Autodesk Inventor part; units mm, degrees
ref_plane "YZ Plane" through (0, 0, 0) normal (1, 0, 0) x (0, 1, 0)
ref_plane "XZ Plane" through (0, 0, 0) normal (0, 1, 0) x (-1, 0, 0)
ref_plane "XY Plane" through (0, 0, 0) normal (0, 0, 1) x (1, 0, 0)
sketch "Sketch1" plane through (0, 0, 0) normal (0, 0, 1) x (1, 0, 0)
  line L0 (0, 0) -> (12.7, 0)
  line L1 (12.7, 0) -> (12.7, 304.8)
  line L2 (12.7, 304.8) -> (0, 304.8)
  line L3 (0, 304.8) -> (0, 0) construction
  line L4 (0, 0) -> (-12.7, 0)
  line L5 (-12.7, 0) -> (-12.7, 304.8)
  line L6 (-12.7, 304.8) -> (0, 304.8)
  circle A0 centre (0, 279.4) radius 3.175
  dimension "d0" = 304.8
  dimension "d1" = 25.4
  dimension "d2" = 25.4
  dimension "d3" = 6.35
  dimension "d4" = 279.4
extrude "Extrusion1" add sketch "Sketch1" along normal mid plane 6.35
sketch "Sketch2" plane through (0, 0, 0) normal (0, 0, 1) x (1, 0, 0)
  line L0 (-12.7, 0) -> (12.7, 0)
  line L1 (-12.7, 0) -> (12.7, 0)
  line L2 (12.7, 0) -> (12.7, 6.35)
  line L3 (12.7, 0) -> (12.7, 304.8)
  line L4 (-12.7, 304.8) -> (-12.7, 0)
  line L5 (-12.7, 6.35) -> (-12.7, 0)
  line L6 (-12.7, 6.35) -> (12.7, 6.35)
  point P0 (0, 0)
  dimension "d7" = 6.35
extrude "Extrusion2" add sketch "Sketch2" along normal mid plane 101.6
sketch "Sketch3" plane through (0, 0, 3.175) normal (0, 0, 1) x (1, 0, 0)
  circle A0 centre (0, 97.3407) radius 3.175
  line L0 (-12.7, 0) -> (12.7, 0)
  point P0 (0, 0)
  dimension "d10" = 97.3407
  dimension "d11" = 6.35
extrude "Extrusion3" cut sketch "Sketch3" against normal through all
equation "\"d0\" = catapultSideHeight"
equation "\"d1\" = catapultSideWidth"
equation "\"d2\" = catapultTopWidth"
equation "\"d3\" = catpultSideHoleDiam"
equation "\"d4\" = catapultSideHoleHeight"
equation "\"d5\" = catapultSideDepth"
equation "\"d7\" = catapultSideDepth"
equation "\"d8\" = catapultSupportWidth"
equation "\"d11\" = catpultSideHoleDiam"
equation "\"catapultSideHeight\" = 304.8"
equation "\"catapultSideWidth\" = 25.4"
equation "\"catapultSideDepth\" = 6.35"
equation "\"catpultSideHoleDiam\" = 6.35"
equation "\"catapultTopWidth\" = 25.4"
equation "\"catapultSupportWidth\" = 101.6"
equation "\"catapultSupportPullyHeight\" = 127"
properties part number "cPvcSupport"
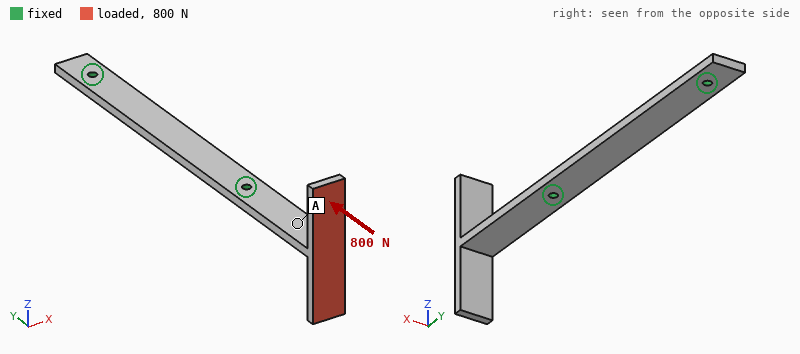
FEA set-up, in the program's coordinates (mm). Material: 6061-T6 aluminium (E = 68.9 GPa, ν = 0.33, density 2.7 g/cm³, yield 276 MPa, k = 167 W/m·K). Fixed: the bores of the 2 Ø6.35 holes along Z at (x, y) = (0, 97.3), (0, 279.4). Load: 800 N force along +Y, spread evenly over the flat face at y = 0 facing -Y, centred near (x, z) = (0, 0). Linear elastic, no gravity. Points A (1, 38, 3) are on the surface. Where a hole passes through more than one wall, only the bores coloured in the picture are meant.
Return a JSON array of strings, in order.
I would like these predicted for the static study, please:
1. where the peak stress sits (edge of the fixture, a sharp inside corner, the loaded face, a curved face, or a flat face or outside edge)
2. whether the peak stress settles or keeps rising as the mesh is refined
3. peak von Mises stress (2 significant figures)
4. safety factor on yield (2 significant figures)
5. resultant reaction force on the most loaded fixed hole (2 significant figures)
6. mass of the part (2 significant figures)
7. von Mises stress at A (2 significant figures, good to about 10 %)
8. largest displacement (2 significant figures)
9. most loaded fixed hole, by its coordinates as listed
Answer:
["the loaded face", "settles", "48 MPa", "5.8", "780 N", "170 g", "4.9 MPa", "0.17 mm", "(0, 97.3)"]
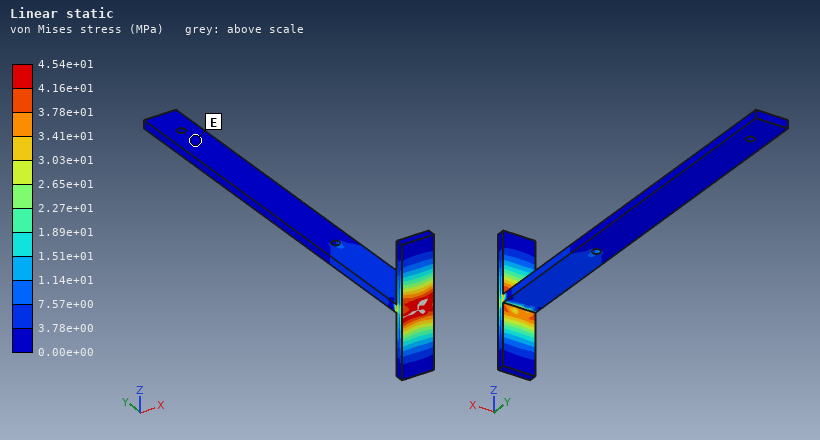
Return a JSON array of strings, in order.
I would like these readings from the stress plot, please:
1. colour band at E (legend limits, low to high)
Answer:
["0.00e+00 to 3.78e+00 MPa"]
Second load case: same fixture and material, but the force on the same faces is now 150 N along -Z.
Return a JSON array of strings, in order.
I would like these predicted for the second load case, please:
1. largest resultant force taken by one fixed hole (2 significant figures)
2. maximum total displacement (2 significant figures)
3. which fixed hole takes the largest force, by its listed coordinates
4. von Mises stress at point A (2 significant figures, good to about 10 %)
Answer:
["150 N", "1.5 mm", "(0, 97.3)", "33 MPa"]
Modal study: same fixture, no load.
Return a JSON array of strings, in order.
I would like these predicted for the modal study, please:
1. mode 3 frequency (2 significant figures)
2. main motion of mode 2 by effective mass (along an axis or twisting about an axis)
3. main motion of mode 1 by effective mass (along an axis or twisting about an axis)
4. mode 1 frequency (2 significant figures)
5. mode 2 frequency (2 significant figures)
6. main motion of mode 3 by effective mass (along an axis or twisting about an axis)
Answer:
["790 Hz", "twisting about Y", "along Z", "240 Hz", "580 Hz", "along X"]
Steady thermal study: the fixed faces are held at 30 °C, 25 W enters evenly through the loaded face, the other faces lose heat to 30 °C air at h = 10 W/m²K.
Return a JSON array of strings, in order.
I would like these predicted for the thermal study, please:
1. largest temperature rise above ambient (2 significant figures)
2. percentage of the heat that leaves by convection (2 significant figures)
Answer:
["80 K", "21 %"]
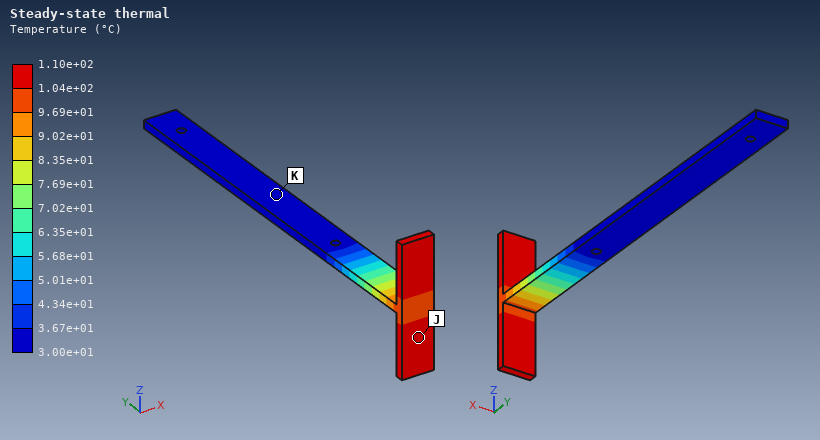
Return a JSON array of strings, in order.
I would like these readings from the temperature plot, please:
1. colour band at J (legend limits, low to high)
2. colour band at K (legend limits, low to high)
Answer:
["1.04e+02 to 1.10e+02 °C", "3.00e+01 to 3.67e+01 °C"]
